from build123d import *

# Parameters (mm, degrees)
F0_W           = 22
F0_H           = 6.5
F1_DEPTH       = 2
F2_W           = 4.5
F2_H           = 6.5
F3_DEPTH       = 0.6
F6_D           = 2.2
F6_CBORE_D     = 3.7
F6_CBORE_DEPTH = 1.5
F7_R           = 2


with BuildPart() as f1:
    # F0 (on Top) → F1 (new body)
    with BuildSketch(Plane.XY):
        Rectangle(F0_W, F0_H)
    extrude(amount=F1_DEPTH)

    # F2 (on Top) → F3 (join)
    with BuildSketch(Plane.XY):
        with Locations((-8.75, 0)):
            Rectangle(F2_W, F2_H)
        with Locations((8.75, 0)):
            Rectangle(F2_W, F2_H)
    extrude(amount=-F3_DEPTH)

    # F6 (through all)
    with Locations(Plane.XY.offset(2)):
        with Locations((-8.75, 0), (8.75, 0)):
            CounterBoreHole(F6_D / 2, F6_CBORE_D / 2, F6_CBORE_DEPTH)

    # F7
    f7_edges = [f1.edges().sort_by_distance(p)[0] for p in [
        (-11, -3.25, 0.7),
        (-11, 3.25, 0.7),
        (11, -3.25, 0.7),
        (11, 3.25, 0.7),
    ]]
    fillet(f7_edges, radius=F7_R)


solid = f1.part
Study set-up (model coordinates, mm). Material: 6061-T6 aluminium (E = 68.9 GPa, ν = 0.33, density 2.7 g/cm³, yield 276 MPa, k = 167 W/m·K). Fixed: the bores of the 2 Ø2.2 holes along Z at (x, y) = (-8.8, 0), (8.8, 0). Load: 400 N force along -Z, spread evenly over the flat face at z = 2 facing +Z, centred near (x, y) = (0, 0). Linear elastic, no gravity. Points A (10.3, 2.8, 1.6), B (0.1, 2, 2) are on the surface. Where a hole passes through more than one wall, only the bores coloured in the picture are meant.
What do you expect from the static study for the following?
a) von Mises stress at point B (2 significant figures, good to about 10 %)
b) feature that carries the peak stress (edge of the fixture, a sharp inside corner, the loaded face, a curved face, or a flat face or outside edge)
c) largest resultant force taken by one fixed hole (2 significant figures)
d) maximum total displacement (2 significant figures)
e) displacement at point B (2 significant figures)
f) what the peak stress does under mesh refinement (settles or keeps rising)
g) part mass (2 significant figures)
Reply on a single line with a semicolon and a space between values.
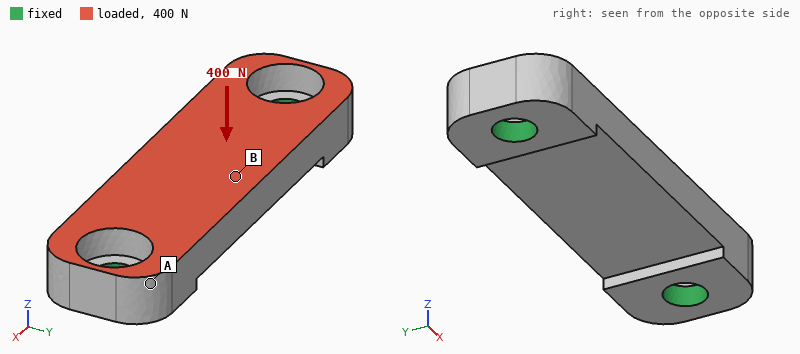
72 MPa; edge of the fixture; 280 N; 20 µm; 19 µm; keeps rising; 0.73 g
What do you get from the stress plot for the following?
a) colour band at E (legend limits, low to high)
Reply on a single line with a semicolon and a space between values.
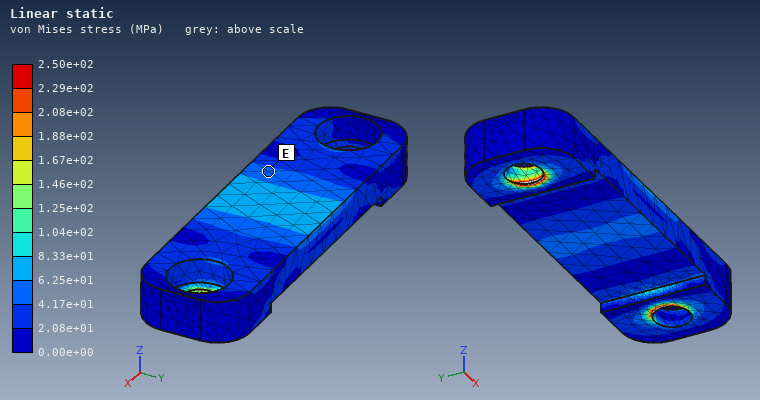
4.17e+01 to 6.25e+01 MPa
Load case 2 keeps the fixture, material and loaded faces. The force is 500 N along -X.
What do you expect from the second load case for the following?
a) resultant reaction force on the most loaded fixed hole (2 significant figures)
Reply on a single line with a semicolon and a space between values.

250 N
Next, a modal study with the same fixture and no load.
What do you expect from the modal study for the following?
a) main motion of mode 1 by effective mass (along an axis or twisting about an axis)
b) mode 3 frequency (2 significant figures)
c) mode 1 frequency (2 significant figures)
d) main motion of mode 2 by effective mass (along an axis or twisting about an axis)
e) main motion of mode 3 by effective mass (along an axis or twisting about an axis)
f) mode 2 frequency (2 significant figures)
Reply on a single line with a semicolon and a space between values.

along Z; 55 kHz; 32 kHz; along Y; along Y; 38 kHz
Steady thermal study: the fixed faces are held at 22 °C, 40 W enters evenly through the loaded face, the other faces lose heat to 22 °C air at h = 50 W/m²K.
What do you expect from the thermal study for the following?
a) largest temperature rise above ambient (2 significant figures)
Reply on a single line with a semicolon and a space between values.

48 K
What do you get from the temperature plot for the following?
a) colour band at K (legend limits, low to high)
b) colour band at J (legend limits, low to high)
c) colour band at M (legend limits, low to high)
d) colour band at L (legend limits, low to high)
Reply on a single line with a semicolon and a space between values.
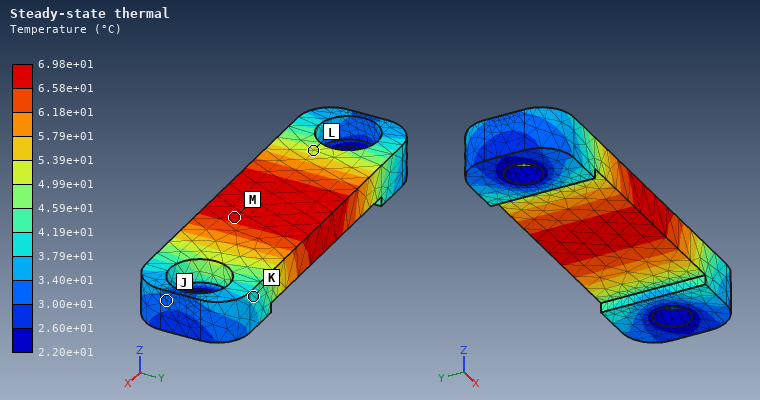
3.79e+01 to 4.19e+01 °C; 3.00e+01 to 3.40e+01 °C; 6.58e+01 to 6.98e+01 °C; 4.99e+01 to 5.39e+01 °C
